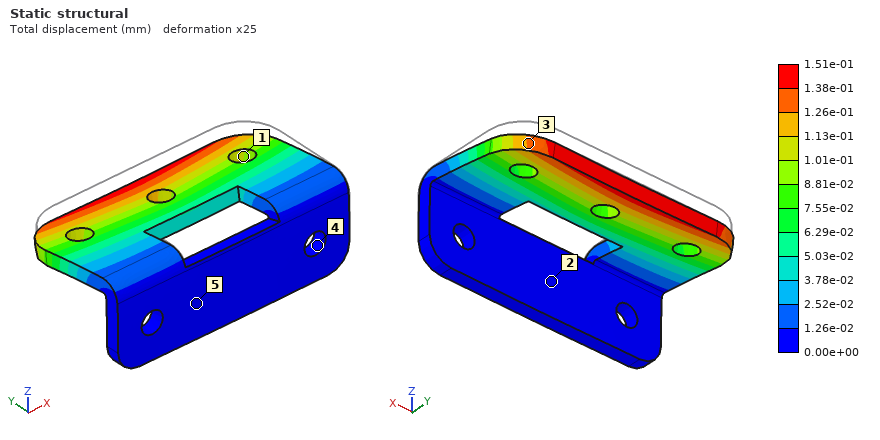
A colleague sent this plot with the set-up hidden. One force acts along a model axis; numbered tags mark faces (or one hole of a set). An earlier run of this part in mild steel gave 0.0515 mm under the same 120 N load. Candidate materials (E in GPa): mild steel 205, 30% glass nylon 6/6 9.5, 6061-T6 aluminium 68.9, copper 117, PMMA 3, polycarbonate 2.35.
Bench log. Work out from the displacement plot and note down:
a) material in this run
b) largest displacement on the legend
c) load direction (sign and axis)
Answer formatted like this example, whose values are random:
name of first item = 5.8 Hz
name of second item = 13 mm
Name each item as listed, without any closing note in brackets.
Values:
material in this run = 6061-T6 aluminium
largest displacement on the legend = 1.51e-01 mm
load direction = -Z
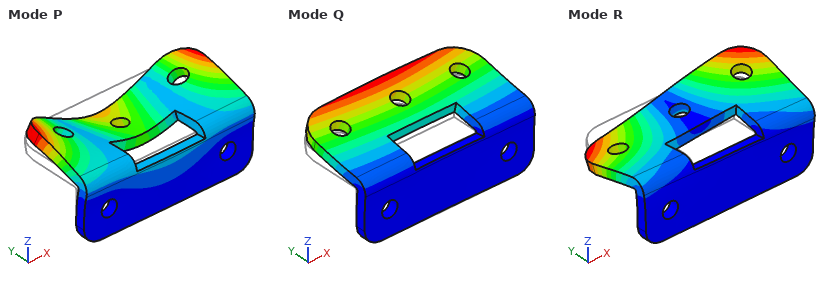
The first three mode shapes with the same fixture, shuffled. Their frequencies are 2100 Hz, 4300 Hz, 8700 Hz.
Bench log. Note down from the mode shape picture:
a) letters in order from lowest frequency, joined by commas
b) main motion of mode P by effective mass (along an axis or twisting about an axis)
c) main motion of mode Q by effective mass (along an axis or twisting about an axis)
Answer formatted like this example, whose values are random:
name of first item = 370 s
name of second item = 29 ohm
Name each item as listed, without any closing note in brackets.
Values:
letters in order from lowest frequency, joined by commas = Q, R, P
main motion of mode P by effective mass = along Y
main motion of mode Q by effective mass = along Z
